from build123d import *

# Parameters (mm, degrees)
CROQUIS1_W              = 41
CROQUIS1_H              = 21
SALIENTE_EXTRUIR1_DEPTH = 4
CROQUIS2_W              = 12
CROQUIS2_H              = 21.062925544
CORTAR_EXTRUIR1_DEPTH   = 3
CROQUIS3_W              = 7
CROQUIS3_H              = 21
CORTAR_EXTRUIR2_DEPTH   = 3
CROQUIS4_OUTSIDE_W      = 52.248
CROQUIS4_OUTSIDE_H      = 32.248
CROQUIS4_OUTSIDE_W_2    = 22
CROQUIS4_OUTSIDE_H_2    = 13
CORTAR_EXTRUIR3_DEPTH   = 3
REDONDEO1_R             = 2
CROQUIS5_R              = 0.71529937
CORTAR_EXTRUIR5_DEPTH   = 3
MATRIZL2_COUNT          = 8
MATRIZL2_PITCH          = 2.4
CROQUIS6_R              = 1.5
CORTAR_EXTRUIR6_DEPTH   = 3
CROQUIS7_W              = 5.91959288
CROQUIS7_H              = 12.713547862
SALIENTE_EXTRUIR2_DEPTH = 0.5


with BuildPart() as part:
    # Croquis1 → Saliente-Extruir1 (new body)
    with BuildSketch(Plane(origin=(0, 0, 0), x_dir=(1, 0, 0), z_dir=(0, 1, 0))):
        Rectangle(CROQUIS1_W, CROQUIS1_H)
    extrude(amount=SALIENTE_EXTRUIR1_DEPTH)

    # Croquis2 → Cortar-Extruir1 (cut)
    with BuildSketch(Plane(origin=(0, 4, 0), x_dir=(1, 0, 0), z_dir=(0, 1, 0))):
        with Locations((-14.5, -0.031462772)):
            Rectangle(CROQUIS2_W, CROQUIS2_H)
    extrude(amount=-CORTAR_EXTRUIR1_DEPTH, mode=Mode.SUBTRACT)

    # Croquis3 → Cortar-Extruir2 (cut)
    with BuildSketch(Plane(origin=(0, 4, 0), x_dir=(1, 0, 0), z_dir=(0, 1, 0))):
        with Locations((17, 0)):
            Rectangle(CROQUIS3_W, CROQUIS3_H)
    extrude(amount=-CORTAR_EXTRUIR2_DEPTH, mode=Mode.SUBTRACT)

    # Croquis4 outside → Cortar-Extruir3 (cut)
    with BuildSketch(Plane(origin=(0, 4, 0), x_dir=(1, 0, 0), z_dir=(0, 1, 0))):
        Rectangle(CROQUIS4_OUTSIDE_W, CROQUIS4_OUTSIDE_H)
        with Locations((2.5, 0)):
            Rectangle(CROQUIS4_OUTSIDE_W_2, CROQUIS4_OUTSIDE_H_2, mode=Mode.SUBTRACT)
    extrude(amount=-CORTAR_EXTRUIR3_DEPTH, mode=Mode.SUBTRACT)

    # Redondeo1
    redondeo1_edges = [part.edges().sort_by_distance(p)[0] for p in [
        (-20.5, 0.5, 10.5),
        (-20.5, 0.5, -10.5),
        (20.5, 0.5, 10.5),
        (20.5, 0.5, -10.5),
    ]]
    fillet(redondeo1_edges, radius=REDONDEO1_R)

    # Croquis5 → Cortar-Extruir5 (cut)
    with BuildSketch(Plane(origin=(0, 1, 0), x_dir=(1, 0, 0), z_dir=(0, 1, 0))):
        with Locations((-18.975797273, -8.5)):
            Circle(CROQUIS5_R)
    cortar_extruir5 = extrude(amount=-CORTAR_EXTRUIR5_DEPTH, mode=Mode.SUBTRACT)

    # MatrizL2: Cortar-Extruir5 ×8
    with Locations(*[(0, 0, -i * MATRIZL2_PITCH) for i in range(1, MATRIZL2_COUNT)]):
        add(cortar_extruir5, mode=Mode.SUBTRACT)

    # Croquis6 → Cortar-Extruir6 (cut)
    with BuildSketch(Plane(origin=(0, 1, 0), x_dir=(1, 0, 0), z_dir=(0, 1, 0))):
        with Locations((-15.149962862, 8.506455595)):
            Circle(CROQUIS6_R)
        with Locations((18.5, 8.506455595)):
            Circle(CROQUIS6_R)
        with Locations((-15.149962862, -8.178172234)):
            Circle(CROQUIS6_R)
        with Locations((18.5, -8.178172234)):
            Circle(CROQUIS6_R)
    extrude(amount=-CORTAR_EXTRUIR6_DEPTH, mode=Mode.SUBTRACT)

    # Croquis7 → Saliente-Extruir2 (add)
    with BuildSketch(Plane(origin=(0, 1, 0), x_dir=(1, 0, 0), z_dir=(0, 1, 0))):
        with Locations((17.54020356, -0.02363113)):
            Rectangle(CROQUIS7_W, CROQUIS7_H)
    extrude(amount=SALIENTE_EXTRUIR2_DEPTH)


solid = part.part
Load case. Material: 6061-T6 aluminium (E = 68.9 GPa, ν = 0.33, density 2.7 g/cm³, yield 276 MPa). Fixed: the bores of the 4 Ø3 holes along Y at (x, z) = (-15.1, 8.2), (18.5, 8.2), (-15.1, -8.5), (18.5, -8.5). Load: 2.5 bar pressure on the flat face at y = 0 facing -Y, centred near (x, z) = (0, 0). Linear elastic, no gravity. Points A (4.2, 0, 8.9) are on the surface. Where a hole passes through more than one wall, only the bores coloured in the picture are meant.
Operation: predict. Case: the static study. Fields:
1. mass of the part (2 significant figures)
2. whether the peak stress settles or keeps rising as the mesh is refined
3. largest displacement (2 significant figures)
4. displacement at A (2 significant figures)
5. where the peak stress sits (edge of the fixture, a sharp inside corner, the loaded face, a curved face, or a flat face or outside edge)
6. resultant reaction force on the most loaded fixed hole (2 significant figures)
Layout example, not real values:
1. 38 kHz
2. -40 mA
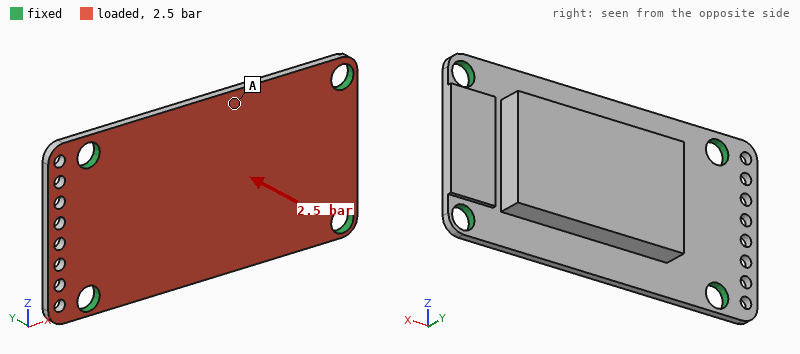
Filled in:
1. 4.6 g
2. keeps rising
3. 24 µm
4. 20 µm
5. edge of the fixture
6. 67 N
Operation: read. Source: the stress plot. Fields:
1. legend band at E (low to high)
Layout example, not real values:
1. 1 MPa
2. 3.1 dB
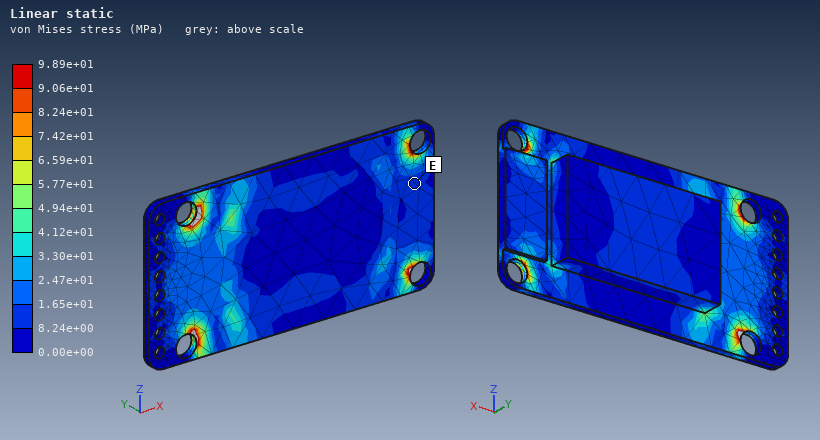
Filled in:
1. 8.24e+00 to 1.65e+01 MPa
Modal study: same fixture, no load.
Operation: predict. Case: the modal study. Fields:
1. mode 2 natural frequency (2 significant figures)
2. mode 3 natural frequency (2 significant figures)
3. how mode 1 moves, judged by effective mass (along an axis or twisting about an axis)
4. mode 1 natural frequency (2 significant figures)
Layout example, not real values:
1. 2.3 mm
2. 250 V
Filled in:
1. 11 kHz
2. 16 kHz
3. along Y
4. 7100 Hz
